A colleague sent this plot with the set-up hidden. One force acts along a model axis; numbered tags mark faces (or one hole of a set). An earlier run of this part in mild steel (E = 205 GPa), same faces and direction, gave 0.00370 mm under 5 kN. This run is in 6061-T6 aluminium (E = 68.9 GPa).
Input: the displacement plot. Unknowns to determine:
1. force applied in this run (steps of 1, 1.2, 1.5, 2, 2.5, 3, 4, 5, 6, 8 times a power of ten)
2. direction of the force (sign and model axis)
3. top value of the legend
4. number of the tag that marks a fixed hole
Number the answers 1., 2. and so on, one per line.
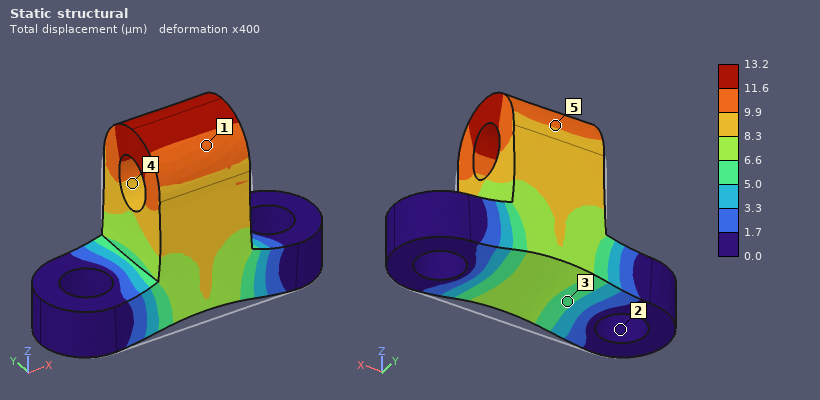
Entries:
1. 6 kN
2. +Z
3. 13.2 µm
4. 2
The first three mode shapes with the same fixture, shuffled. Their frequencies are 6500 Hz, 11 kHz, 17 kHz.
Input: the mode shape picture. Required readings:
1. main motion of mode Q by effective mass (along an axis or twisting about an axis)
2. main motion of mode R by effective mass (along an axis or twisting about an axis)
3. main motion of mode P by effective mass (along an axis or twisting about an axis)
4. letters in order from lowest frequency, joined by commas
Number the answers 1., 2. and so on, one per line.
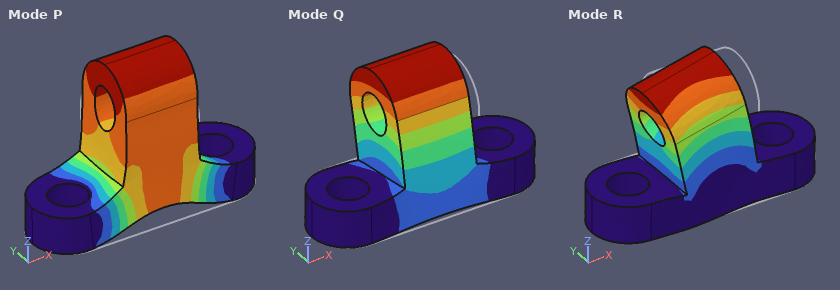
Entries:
1. along Y
2. along X
3. along Z
4. Q, R, P
